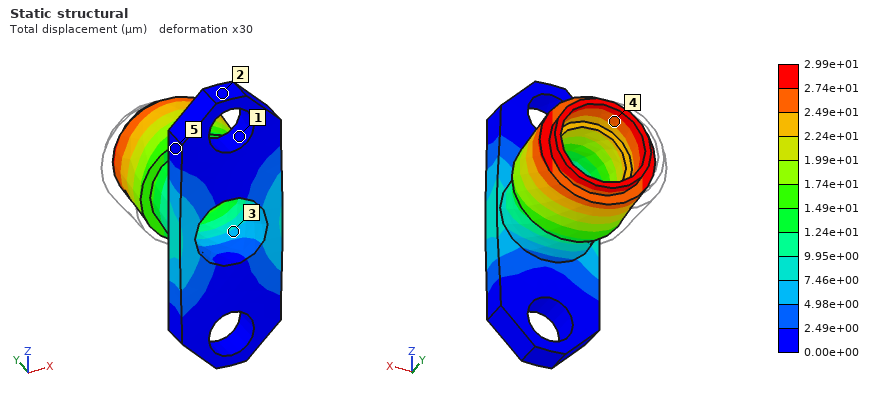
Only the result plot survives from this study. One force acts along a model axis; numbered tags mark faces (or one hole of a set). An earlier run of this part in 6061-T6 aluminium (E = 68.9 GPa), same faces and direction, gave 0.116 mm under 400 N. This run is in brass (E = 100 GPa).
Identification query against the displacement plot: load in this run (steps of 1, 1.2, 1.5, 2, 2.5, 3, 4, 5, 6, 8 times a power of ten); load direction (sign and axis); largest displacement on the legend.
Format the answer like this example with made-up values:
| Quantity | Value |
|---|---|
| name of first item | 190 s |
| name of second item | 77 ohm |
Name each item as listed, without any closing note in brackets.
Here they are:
| Quantity | Value |
|---|---|
| load in this run | 150 N |
| load direction | +X |
| largest displacement on the legend | 2.99e+01 µm |
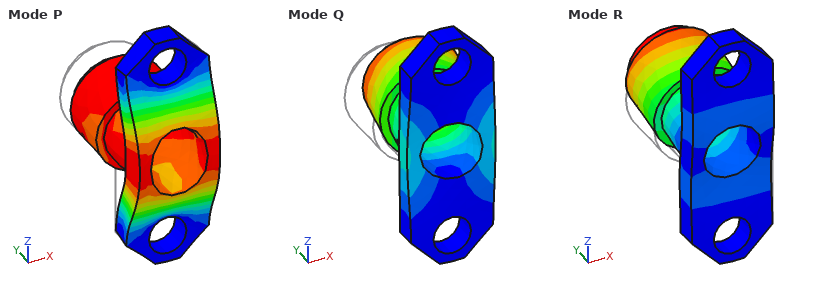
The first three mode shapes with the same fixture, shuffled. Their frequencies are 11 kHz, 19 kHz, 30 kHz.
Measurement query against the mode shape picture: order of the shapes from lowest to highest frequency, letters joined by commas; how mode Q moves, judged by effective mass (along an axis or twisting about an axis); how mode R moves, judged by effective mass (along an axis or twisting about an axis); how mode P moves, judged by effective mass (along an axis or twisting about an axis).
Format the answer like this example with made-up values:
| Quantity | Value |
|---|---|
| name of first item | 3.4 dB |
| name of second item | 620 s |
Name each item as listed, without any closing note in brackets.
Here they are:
| Quantity | Value |
|---|---|
| order of the shapes from lowest to highest frequency, letters joined by commas | Q, R, P |
| how mode Q moves, judged by effective mass | along X |
| how mode R moves, judged by effective mass | along Z |
| how mode P moves, judged by effective mass | along Y |
